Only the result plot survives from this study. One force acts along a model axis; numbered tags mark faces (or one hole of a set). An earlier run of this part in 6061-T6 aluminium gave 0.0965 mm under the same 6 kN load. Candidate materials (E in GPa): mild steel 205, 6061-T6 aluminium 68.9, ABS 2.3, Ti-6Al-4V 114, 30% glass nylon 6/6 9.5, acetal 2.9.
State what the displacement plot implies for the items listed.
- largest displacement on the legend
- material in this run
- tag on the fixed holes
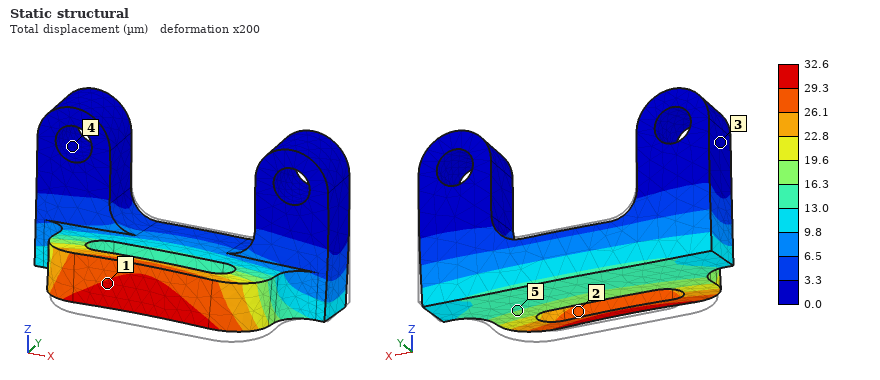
32.6 µm
mild steel
4
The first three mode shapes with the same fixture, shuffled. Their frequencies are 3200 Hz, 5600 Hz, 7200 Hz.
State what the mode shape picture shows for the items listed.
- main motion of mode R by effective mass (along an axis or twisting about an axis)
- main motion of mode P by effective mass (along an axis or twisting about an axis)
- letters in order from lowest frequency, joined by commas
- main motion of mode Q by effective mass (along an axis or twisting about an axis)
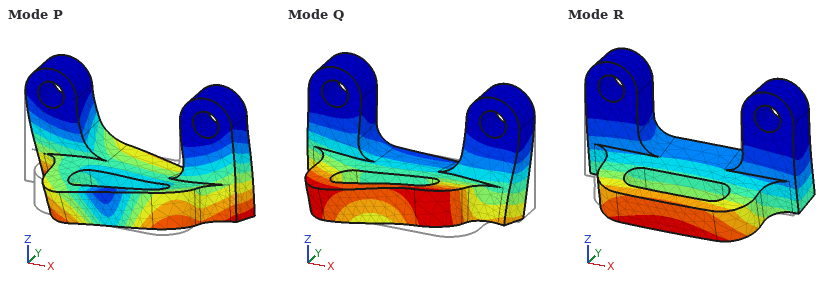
along Y
along X
R, Q, P
along X
